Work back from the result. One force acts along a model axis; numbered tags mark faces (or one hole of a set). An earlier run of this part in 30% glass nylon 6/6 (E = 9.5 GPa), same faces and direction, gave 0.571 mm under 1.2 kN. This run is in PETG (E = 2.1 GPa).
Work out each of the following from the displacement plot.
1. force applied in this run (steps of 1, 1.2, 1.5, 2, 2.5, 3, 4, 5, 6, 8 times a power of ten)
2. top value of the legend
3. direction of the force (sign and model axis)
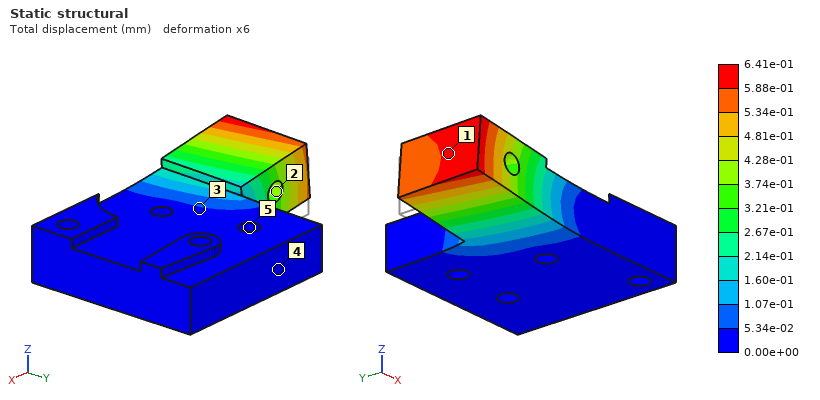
300 N
6.41e-01 mm
+Z
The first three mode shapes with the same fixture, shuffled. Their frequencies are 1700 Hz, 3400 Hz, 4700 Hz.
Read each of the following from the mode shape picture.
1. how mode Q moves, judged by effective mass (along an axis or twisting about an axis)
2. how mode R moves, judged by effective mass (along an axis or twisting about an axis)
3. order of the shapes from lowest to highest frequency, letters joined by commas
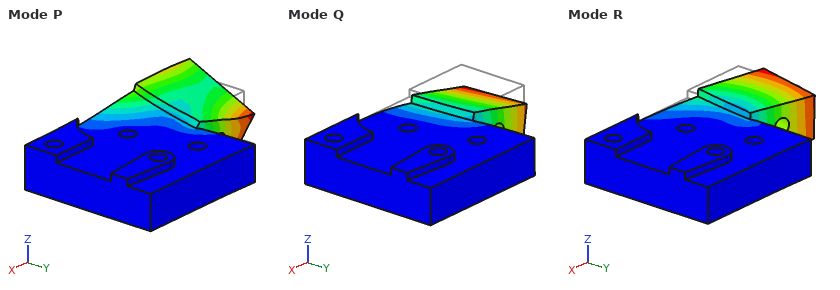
along Z
along Y
Q, R, P
